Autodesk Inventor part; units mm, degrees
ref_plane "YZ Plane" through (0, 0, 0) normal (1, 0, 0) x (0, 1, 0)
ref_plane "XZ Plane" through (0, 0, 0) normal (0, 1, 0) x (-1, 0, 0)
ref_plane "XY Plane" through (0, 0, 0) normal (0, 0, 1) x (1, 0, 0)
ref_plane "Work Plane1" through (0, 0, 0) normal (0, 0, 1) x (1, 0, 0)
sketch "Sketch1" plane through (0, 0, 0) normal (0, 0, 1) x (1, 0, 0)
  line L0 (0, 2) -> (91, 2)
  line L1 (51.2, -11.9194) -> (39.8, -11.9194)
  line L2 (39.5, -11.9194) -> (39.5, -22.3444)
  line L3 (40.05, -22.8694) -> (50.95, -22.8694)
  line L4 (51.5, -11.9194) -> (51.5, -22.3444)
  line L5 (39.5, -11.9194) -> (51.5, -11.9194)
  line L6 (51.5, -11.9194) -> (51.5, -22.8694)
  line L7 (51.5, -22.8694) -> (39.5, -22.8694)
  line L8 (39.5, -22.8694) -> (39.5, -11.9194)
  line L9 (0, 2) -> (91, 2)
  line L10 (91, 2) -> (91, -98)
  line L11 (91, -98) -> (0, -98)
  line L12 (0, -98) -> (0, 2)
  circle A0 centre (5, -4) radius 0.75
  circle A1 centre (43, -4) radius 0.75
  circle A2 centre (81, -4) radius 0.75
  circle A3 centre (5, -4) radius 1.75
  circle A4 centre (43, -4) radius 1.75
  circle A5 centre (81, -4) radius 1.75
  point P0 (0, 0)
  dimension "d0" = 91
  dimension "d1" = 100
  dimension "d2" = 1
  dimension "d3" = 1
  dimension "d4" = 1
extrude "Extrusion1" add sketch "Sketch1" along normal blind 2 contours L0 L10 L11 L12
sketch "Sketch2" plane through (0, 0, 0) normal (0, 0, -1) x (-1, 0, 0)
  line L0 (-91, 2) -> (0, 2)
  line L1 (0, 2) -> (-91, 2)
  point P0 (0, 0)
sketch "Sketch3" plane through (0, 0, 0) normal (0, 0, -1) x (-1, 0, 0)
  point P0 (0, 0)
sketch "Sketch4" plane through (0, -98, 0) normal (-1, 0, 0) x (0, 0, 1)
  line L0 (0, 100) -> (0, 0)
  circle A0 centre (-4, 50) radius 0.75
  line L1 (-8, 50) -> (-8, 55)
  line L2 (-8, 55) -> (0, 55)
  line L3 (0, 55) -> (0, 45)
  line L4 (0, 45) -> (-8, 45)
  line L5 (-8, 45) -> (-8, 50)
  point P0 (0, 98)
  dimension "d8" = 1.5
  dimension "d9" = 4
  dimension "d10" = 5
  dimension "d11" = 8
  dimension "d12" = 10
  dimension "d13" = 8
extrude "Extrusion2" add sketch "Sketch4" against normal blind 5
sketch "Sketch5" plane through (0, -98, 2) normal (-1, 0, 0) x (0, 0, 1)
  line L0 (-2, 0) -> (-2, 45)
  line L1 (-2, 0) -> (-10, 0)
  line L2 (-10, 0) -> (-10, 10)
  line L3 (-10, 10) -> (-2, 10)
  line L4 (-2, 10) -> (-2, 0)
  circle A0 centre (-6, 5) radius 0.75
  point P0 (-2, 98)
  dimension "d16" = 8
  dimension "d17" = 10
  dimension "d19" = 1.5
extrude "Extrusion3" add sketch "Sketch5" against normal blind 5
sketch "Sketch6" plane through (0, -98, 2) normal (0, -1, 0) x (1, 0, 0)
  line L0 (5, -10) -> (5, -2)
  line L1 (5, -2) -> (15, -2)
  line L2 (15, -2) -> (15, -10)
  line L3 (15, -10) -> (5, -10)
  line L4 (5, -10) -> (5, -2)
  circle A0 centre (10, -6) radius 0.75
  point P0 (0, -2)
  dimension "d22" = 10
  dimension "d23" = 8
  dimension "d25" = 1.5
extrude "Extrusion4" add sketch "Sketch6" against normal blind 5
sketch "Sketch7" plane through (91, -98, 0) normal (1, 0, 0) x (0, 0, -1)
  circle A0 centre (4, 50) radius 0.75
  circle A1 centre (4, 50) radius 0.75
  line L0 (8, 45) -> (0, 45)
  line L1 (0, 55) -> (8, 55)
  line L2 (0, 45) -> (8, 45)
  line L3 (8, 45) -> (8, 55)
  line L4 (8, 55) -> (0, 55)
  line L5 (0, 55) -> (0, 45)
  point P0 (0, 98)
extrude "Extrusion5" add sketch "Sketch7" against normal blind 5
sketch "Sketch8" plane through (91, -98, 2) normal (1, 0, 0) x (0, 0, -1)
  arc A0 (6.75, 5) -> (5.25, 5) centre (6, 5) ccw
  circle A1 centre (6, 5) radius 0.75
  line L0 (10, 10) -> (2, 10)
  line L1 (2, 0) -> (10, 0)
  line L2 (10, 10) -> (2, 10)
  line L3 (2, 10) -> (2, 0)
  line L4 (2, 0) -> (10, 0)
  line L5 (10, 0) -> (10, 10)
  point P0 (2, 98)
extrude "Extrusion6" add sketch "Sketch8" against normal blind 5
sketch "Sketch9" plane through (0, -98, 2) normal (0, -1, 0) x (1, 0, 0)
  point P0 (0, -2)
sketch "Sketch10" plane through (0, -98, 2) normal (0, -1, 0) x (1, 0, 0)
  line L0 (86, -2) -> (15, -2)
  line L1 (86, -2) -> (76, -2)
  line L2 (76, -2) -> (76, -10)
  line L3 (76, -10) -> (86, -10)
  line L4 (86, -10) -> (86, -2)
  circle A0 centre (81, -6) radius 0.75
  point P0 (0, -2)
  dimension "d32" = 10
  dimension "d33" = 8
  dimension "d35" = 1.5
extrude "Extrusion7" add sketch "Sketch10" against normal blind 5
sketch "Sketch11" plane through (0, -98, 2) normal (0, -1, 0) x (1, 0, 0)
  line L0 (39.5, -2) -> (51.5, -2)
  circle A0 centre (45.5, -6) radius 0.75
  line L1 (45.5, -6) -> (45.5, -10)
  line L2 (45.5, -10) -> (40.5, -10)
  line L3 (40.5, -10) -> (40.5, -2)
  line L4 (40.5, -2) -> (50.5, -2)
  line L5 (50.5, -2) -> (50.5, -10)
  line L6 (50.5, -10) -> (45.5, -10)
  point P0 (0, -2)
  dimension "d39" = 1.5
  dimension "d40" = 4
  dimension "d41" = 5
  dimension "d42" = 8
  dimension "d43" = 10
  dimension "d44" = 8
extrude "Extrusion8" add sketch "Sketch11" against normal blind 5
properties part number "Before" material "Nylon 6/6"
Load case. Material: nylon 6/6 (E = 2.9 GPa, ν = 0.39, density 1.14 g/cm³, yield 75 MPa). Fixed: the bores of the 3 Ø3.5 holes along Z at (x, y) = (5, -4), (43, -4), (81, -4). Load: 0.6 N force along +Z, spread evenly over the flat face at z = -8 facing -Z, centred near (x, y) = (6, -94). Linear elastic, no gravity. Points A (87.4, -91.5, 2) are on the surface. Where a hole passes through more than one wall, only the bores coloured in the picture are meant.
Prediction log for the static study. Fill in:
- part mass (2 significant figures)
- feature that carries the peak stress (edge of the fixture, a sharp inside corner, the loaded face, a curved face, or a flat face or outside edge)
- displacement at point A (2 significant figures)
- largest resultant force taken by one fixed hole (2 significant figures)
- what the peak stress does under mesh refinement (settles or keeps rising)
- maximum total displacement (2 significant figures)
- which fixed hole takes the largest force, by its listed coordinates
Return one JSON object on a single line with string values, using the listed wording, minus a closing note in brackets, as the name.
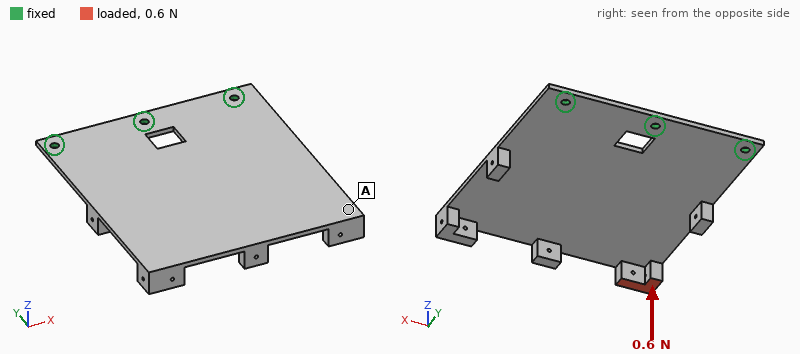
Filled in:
{"part mass": "24 g", "feature that carries the peak stress": "edge of the fixture", "displacement at point A": "0.64 mm", "largest resultant force taken by one fixed hole": "0.47 N", "what the peak stress does under mesh refinement": "keeps rising", "maximum total displacement": "1.3 mm", "which fixed hole takes the largest force, by its listed coordinates": "(5, -4)"}
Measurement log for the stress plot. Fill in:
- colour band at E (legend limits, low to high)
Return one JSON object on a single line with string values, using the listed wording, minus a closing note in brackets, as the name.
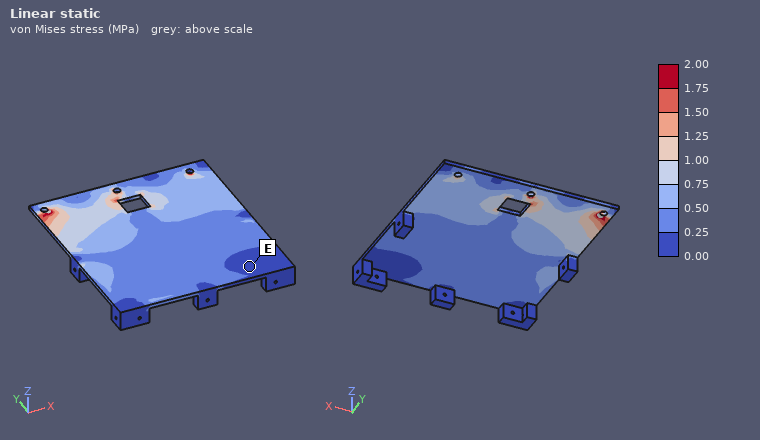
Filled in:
{"colour band at E": "0.00 to 0.25 MPa"}
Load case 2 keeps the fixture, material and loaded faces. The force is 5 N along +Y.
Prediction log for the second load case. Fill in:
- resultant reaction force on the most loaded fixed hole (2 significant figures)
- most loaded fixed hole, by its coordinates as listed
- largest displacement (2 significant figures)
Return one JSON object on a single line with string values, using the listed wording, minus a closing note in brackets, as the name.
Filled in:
{"resultant reaction force on the most loaded fixed hole": "4.1 N", "most loaded fixed hole, by its coordinates as listed": "(5, -4)", "largest displacement": "1.5 mm"}
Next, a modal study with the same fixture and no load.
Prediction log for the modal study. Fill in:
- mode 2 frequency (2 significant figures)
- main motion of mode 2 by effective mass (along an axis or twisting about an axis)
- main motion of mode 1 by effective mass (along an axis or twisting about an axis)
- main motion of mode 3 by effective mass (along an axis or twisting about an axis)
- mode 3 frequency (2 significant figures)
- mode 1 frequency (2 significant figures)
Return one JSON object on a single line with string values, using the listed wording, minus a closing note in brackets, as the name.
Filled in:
{"mode 2 frequency": "120 Hz", "main motion of mode 2 by effective mass": "twisting about Y", "main motion of mode 1 by effective mass": "along Z", "main motion of mode 3 by effective mass": "along Z", "mode 3 frequency": "310 Hz", "mode 1 frequency": "46 Hz"}
